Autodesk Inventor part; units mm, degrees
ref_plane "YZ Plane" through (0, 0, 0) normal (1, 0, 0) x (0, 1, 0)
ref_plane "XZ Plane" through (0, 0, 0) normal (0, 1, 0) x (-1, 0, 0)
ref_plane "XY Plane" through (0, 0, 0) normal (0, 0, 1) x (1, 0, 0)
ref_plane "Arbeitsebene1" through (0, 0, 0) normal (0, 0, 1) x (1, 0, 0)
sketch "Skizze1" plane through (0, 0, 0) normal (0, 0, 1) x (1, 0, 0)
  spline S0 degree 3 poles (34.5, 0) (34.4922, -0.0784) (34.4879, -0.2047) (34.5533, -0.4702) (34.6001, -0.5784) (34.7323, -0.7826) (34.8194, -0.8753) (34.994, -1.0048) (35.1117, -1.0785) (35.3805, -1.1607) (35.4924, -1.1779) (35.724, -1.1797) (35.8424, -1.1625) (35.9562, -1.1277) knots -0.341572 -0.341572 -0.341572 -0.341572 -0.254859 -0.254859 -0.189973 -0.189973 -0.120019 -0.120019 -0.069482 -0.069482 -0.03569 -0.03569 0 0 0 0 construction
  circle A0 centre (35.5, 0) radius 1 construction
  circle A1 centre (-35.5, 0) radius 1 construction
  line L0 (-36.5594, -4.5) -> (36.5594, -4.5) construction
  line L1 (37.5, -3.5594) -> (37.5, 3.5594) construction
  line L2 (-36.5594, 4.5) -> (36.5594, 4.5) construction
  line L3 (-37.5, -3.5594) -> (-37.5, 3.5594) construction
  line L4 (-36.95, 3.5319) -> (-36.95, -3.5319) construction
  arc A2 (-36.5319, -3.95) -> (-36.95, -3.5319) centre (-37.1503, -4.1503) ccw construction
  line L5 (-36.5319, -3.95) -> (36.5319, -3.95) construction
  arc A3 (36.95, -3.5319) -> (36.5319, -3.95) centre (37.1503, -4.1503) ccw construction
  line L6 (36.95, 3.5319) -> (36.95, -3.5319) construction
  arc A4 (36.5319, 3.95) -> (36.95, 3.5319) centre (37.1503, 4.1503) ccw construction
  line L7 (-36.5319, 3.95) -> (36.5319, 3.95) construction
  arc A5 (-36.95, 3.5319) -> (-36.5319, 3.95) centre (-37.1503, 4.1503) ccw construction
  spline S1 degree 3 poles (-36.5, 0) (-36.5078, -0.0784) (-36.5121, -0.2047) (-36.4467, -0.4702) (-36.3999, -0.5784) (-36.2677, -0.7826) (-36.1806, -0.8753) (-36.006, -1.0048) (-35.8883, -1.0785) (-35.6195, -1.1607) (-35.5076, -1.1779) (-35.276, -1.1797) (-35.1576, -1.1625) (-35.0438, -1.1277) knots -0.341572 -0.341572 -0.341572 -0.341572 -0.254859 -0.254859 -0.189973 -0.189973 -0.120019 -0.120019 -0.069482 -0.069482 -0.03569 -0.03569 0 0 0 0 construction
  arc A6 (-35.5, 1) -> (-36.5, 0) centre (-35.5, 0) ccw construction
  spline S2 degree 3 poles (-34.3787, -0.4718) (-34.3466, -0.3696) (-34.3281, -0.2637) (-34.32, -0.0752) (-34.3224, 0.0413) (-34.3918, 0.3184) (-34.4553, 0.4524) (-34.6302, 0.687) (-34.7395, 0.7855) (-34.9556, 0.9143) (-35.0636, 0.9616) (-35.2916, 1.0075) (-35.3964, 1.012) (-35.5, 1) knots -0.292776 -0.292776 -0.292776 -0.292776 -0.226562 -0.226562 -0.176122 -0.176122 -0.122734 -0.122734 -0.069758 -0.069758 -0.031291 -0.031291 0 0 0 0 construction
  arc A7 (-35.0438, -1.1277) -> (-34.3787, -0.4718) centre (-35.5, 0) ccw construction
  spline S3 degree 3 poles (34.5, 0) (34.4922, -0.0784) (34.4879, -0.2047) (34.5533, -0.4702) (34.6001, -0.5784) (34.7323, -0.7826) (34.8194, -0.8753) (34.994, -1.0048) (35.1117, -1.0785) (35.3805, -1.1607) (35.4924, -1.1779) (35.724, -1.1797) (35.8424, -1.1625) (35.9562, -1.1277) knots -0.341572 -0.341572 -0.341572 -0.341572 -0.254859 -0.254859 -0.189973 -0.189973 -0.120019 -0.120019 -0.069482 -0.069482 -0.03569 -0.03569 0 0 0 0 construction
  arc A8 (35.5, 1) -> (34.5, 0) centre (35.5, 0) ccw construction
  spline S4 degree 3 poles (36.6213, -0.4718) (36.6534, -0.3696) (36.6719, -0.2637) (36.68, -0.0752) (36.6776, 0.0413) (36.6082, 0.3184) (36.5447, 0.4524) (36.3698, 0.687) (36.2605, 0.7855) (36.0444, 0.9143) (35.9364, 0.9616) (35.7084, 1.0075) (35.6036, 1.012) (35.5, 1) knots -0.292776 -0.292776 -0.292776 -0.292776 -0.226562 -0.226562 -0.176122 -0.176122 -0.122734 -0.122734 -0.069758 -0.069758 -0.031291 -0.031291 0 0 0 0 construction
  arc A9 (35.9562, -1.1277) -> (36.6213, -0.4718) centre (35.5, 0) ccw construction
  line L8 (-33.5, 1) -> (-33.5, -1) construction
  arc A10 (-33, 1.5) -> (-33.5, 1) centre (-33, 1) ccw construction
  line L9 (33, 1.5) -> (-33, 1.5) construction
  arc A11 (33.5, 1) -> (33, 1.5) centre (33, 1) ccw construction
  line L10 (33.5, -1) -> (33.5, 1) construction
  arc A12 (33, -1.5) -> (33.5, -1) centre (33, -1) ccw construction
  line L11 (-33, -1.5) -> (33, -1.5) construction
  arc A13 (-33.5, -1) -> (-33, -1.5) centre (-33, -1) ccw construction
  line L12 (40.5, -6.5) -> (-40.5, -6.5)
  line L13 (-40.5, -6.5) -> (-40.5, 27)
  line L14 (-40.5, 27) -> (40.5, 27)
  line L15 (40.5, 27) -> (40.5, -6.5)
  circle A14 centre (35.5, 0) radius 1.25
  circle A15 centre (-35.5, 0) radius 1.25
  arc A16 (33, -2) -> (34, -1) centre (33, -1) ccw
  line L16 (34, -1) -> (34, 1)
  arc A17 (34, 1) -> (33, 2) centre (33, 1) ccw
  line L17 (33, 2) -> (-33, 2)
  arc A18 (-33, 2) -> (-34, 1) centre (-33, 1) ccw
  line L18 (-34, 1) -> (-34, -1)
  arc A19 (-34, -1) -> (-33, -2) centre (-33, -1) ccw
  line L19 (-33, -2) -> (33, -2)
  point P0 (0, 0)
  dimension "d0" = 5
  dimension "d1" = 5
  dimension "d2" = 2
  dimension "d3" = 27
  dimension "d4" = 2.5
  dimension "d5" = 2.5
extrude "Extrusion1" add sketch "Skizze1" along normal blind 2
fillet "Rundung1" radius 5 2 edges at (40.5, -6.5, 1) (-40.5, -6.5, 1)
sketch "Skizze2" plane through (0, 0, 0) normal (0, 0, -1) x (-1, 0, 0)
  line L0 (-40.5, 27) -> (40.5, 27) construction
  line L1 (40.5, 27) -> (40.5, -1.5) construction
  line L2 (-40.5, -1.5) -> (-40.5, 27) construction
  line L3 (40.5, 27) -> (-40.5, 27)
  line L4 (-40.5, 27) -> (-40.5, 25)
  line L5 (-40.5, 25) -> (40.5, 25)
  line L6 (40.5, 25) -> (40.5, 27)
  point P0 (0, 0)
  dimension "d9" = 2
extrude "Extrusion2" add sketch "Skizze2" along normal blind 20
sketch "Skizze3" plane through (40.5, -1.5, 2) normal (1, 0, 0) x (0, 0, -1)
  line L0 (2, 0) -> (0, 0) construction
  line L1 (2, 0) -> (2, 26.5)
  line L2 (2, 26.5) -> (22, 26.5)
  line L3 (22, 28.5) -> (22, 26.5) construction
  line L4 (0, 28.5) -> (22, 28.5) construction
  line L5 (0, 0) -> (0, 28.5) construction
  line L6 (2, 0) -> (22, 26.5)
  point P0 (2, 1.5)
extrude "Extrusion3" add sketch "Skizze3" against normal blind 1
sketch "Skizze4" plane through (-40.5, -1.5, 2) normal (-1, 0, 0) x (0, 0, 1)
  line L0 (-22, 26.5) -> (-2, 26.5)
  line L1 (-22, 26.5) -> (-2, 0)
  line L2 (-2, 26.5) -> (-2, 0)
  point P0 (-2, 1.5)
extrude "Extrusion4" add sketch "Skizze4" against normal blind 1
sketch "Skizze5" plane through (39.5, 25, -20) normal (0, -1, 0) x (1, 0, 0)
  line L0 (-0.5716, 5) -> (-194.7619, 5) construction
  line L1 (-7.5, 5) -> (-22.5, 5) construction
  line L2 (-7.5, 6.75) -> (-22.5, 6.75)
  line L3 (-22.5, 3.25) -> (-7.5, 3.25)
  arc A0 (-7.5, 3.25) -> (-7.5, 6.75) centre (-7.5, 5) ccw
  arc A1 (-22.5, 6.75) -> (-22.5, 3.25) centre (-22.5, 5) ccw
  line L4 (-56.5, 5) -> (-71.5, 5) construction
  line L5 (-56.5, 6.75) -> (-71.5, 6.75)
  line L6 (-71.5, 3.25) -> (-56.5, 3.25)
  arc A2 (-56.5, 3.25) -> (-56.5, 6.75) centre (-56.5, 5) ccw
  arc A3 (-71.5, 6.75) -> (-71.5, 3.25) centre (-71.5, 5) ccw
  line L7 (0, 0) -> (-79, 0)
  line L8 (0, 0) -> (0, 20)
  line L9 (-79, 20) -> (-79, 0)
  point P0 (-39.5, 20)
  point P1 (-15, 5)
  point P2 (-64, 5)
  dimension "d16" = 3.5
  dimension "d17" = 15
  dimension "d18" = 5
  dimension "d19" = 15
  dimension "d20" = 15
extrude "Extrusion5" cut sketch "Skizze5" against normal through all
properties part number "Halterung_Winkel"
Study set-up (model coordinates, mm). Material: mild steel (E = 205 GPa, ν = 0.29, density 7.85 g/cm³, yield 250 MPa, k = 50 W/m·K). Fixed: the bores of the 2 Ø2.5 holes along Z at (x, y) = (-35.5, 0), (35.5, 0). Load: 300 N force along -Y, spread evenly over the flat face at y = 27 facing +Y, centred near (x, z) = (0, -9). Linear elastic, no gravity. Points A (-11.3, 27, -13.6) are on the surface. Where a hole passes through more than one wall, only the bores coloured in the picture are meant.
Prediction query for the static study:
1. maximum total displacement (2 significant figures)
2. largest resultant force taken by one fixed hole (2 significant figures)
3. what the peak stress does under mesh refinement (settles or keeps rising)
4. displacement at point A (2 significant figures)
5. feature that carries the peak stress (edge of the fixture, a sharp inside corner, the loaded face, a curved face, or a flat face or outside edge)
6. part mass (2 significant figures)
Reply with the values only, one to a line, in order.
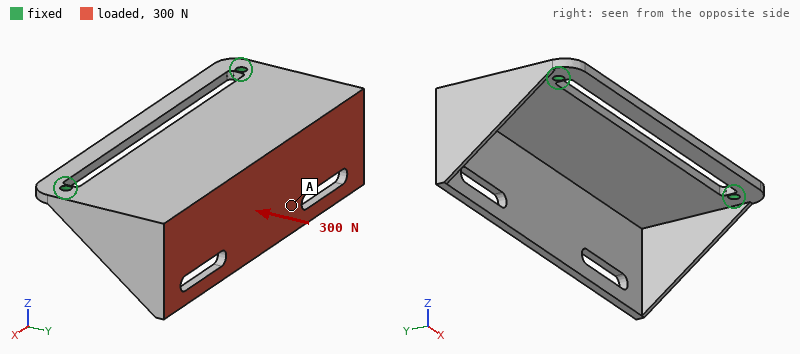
0.21 mm
170 N
keeps rising
0.17 mm
edge of the fixture
66 g
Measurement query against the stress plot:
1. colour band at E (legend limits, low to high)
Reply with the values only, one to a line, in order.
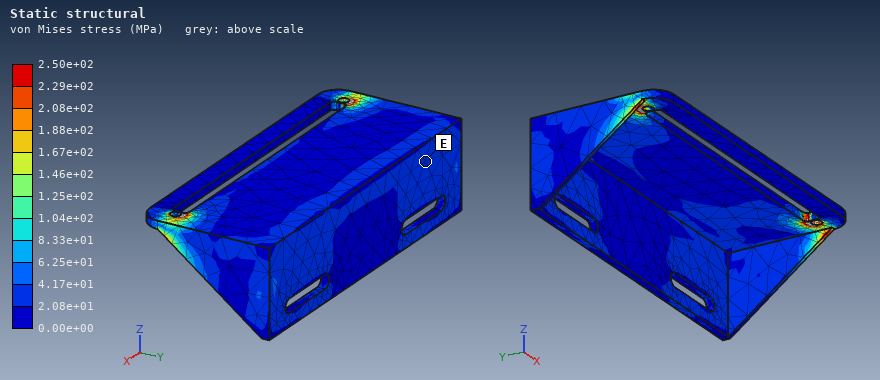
2.08e+01 to 4.17e+01 MPa
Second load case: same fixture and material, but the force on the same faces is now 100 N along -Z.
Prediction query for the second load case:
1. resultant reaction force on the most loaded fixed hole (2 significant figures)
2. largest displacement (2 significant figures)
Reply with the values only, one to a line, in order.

52 N
0.14 mm
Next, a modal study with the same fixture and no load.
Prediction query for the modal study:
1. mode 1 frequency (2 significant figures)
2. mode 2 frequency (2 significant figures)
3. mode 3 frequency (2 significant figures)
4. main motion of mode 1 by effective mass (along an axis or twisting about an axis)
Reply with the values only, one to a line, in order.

800 Hz
1600 Hz
2000 Hz
along Z
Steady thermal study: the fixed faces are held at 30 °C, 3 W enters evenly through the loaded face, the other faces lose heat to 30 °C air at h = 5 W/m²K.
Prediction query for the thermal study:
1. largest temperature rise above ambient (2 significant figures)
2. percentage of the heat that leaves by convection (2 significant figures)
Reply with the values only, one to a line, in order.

22 K
19 %
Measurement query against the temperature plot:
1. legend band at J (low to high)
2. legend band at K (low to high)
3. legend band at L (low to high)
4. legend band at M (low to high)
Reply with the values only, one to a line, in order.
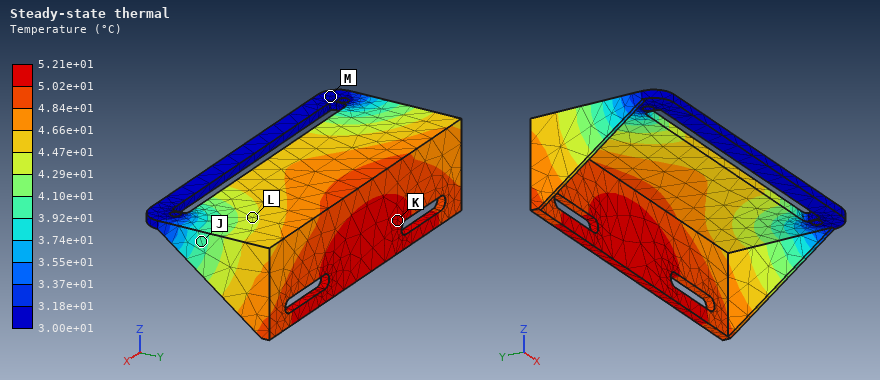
3.92e+01 to 4.10e+01 °C
5.02e+01 to 5.21e+01 °C
4.29e+01 to 4.47e+01 °C
3.00e+01 to 3.18e+01 °C
